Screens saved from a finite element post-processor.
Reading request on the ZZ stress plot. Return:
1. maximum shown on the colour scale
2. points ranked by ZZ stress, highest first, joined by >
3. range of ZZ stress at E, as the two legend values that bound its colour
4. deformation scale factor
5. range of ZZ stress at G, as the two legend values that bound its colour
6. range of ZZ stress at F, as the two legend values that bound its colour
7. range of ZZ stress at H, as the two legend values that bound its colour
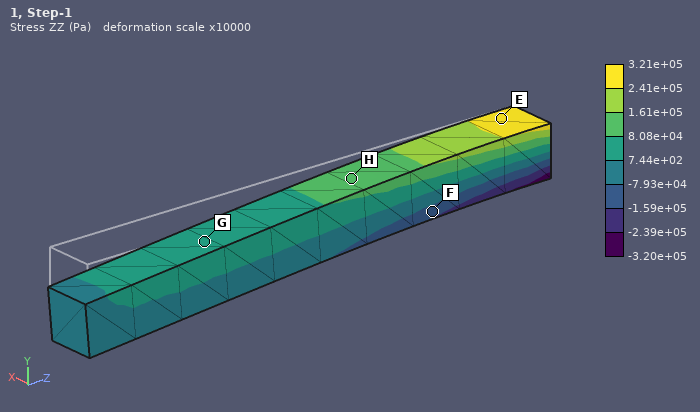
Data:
3.21e+05 Pa
E > H > G > F
2.41e+05 to 3.21e+05 Pa
10000
7.44e+02 to 8.08e+04 Pa
-1.59e+05 to -7.93e+04 Pa
8.08e+04 to 1.61e+05 Pa
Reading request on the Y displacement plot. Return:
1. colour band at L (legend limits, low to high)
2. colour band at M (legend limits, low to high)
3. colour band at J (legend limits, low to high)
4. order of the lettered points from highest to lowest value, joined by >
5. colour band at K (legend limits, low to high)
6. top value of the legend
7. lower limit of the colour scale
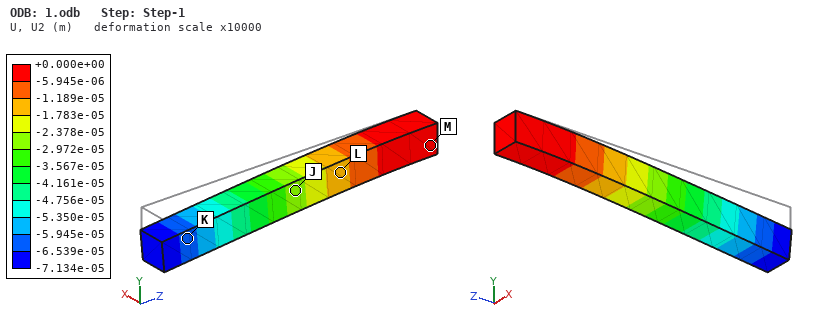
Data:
-1.783e-05 to -1.189e-05 m
-5.945e-06 to +0.000e+00 m
-2.972e-05 to -2.378e-05 m
M > L > J > K
-6.539e-05 to -5.945e-05 m
+0.000e+00 m
-7.134e-05 m
